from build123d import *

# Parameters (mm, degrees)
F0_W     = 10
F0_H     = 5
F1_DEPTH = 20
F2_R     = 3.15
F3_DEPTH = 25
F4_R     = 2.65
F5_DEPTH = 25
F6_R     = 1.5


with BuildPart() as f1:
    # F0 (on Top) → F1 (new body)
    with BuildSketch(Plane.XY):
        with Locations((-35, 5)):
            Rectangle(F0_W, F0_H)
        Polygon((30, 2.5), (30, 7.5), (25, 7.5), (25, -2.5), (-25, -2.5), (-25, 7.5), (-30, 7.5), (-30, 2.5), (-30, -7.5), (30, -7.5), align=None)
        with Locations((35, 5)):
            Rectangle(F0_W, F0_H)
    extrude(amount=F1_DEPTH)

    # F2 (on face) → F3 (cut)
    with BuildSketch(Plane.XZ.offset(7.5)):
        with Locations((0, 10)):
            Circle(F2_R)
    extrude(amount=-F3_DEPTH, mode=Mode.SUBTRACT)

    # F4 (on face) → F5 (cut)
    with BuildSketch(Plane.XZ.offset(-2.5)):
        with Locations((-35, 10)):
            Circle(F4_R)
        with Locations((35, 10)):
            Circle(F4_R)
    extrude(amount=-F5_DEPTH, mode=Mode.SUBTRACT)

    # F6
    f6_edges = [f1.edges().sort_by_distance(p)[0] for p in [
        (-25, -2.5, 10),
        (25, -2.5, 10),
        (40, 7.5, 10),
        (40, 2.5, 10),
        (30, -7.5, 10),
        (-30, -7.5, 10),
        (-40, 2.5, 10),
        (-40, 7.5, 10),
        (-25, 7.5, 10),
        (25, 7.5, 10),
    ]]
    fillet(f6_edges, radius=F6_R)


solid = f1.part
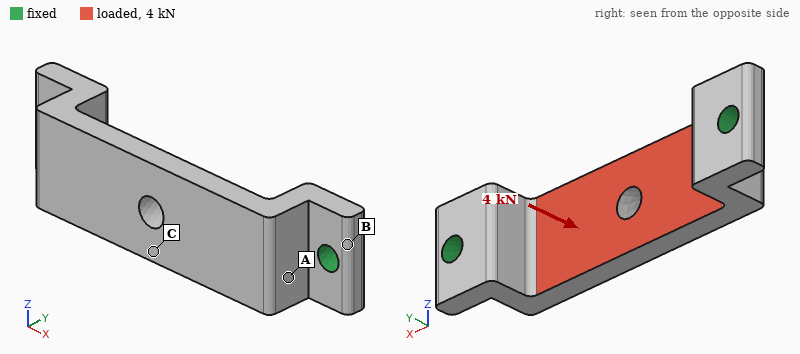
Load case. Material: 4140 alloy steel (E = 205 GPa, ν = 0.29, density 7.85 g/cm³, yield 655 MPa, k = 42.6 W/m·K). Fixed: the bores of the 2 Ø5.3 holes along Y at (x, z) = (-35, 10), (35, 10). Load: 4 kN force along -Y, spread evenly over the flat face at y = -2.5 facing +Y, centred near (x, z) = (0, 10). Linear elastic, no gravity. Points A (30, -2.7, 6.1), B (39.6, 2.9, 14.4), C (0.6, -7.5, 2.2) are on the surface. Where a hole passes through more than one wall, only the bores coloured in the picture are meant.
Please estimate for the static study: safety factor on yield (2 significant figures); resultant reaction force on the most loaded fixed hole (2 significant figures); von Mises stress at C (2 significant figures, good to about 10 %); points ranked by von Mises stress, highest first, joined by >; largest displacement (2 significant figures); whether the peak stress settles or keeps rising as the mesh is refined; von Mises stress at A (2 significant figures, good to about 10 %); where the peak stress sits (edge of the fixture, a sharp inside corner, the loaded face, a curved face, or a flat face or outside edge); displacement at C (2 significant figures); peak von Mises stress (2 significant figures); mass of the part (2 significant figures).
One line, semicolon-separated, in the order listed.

1.9; 3.4 kN; 190 MPa; C > A > B; 67 µm; settles; 83 MPa; a curved face; 66 µm; 350 MPa; 75 g
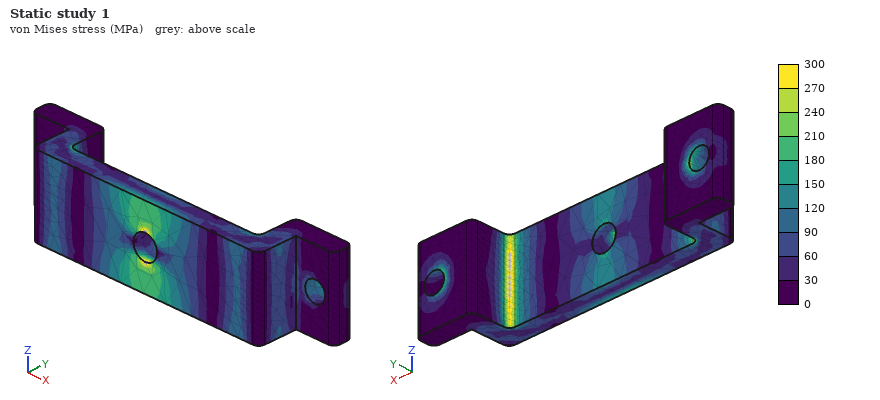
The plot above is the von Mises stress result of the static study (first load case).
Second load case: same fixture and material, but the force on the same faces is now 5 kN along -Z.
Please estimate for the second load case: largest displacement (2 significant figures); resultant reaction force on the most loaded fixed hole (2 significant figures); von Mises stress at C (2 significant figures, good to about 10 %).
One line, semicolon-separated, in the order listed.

44 µm; 2.5 kN; 93 MPa
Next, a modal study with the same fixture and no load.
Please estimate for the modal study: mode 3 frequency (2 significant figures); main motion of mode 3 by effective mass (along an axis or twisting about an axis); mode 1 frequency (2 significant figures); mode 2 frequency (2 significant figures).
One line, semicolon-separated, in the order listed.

9100 Hz; along X; 7500 Hz; 7600 Hz
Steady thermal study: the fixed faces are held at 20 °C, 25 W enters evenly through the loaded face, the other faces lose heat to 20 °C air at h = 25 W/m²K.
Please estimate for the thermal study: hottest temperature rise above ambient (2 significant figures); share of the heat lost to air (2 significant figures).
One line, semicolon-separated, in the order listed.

74 K; 14 %
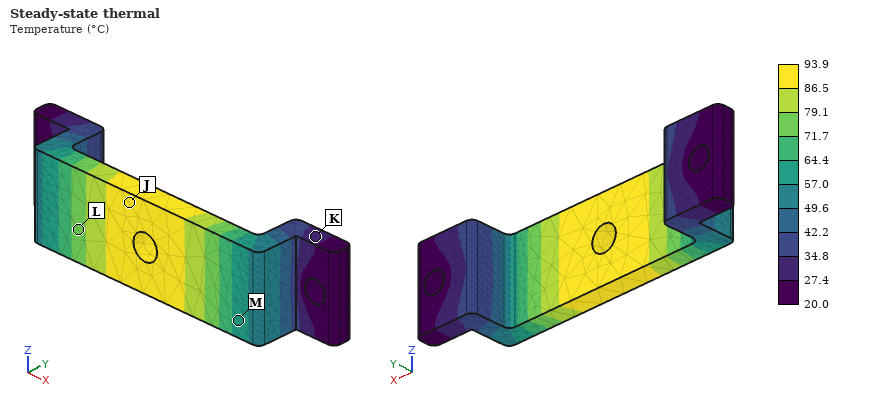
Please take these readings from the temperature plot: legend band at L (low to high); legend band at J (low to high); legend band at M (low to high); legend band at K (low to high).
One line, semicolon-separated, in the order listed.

71.7 to 79.1 °C; 86.5 to 93.9 °C; 57.0 to 64.4 °C; 27.4 to 34.8 °C
